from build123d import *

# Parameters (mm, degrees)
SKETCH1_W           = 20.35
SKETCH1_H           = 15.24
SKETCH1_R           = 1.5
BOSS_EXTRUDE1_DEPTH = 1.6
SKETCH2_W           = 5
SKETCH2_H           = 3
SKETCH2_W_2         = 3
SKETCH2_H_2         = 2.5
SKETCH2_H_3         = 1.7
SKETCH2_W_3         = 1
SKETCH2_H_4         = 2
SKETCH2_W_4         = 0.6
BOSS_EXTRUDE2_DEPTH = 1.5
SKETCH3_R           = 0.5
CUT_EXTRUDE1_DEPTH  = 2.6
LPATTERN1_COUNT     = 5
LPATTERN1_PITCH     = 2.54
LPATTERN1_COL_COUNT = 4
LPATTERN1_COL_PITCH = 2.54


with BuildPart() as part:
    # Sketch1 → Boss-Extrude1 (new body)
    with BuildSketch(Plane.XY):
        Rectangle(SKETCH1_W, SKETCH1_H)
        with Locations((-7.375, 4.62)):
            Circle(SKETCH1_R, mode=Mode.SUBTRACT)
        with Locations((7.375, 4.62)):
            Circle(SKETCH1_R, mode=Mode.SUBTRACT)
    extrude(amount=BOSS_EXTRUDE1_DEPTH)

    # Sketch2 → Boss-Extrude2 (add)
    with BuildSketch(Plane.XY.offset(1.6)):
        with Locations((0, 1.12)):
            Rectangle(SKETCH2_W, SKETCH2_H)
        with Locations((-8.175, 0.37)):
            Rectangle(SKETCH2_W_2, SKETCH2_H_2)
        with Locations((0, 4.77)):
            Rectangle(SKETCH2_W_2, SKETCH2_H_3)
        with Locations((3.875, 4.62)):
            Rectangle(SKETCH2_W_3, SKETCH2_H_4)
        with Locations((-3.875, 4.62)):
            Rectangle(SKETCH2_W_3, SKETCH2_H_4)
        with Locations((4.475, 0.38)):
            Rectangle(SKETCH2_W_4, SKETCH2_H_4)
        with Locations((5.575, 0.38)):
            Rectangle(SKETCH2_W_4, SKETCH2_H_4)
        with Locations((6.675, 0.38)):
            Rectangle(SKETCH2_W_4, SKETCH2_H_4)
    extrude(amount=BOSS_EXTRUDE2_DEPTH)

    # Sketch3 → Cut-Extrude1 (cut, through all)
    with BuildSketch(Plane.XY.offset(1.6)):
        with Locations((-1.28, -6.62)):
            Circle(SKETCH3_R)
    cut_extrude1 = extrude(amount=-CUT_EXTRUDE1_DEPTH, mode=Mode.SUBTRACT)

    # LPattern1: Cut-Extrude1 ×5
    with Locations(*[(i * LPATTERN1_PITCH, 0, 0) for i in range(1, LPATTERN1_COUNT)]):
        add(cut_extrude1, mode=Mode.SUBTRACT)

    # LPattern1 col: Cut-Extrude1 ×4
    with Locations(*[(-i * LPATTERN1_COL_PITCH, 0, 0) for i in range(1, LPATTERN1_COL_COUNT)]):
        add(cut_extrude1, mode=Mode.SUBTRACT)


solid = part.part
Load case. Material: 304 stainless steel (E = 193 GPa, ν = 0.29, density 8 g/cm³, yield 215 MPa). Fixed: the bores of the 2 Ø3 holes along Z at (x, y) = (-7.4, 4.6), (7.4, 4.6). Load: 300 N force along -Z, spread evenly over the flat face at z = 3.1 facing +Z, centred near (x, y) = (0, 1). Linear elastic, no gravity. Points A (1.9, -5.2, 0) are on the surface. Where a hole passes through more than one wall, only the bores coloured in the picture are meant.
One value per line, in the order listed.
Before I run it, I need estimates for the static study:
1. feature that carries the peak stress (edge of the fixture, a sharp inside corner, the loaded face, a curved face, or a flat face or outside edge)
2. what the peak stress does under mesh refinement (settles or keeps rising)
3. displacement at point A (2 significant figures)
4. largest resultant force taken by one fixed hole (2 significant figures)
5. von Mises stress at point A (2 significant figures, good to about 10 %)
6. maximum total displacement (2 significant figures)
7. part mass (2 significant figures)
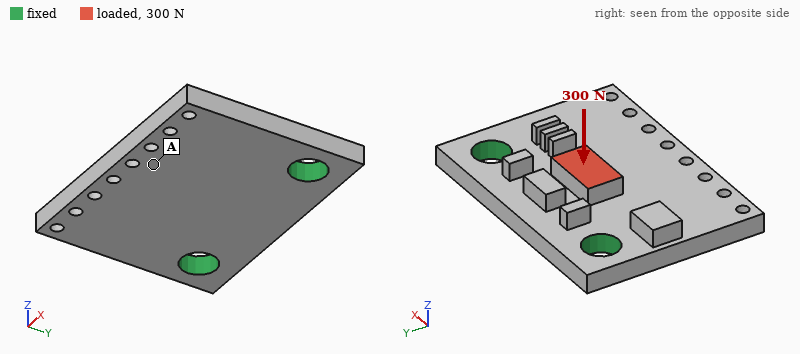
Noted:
edge of the fixture
keeps rising
16 µm
150 N
35 MPa
20 µm
4.1 g
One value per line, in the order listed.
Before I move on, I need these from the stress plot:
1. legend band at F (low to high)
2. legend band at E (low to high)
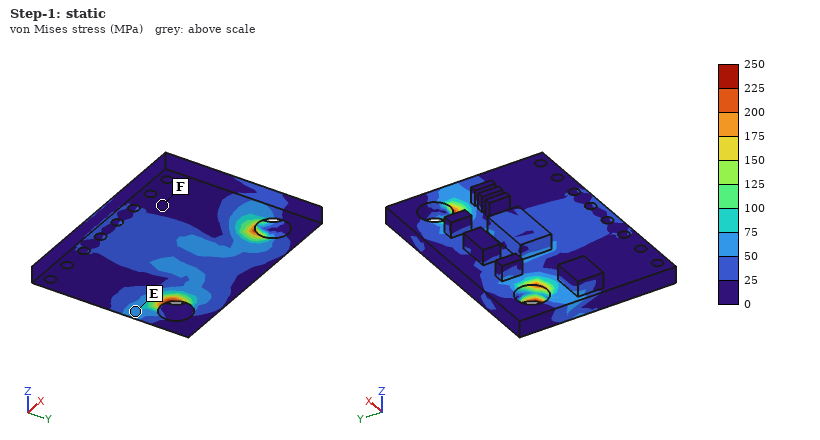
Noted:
0 to 25 MPa
50 to 75 MPa
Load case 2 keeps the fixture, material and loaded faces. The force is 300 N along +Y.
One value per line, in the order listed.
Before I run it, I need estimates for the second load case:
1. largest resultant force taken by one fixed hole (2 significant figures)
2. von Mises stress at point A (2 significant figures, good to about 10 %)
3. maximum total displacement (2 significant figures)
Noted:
160 N
31 MPa
18 µm
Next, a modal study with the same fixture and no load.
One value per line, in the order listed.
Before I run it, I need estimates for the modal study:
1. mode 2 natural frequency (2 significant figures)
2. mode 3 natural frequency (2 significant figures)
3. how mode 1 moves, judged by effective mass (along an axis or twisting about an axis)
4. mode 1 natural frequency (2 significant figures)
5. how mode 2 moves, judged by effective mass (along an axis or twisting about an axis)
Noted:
17 kHz
30 kHz
along Z
9700 Hz
twisting about Y
